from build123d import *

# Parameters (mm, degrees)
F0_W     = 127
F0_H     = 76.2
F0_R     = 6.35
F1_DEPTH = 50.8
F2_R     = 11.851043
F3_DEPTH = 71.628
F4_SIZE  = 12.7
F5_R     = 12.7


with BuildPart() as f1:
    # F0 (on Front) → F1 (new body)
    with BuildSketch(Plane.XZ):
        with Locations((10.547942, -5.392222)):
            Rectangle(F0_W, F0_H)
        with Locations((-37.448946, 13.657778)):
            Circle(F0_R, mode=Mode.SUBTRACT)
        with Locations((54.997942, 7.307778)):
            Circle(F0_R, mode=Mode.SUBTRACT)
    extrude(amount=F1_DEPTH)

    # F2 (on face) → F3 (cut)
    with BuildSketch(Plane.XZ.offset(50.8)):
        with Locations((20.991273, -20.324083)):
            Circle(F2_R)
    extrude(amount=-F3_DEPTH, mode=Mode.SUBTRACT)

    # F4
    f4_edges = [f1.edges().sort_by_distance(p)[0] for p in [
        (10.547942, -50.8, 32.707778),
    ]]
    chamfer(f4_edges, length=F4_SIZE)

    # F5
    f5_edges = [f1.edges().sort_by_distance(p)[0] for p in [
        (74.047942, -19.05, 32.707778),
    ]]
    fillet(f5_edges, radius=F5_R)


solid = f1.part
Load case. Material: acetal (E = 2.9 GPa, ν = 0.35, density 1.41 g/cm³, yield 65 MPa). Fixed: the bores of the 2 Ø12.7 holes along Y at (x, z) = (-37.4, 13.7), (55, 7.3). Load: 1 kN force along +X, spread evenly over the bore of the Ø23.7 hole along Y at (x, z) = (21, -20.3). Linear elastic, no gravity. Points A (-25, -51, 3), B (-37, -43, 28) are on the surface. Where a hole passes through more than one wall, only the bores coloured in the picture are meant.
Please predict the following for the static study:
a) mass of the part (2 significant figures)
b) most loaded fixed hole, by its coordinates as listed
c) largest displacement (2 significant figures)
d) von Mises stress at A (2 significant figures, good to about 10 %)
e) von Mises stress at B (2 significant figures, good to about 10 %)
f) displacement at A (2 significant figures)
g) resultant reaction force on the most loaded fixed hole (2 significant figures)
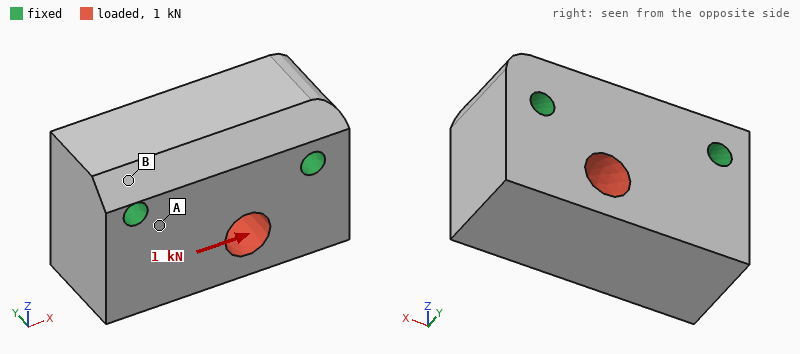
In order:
630 g
(55, 7.3)
11 µm
0.30 MPa
0.12 MPa
1.8 µm
650 N
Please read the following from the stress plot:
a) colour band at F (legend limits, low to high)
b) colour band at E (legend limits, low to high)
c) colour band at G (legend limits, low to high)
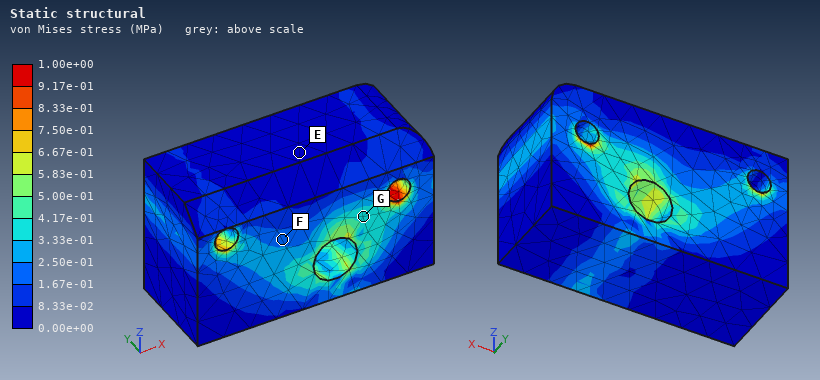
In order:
1.67e-01 to 2.50e-01 MPa
0.00e+00 to 8.33e-02 MPa
3.33e-01 to 4.17e-01 MPa
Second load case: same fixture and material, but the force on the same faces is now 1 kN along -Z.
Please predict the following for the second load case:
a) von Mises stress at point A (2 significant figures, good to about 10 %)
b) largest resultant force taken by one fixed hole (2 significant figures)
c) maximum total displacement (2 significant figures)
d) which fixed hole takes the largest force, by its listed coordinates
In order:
0.34 MPa
650 N
11 µm
(55, 7.3)
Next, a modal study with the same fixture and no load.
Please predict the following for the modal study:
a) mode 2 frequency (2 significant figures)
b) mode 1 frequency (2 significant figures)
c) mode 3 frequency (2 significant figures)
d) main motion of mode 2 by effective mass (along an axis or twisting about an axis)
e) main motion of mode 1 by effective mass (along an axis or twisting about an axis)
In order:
2900 Hz
2100 Hz
3200 Hz
along X
along Y
